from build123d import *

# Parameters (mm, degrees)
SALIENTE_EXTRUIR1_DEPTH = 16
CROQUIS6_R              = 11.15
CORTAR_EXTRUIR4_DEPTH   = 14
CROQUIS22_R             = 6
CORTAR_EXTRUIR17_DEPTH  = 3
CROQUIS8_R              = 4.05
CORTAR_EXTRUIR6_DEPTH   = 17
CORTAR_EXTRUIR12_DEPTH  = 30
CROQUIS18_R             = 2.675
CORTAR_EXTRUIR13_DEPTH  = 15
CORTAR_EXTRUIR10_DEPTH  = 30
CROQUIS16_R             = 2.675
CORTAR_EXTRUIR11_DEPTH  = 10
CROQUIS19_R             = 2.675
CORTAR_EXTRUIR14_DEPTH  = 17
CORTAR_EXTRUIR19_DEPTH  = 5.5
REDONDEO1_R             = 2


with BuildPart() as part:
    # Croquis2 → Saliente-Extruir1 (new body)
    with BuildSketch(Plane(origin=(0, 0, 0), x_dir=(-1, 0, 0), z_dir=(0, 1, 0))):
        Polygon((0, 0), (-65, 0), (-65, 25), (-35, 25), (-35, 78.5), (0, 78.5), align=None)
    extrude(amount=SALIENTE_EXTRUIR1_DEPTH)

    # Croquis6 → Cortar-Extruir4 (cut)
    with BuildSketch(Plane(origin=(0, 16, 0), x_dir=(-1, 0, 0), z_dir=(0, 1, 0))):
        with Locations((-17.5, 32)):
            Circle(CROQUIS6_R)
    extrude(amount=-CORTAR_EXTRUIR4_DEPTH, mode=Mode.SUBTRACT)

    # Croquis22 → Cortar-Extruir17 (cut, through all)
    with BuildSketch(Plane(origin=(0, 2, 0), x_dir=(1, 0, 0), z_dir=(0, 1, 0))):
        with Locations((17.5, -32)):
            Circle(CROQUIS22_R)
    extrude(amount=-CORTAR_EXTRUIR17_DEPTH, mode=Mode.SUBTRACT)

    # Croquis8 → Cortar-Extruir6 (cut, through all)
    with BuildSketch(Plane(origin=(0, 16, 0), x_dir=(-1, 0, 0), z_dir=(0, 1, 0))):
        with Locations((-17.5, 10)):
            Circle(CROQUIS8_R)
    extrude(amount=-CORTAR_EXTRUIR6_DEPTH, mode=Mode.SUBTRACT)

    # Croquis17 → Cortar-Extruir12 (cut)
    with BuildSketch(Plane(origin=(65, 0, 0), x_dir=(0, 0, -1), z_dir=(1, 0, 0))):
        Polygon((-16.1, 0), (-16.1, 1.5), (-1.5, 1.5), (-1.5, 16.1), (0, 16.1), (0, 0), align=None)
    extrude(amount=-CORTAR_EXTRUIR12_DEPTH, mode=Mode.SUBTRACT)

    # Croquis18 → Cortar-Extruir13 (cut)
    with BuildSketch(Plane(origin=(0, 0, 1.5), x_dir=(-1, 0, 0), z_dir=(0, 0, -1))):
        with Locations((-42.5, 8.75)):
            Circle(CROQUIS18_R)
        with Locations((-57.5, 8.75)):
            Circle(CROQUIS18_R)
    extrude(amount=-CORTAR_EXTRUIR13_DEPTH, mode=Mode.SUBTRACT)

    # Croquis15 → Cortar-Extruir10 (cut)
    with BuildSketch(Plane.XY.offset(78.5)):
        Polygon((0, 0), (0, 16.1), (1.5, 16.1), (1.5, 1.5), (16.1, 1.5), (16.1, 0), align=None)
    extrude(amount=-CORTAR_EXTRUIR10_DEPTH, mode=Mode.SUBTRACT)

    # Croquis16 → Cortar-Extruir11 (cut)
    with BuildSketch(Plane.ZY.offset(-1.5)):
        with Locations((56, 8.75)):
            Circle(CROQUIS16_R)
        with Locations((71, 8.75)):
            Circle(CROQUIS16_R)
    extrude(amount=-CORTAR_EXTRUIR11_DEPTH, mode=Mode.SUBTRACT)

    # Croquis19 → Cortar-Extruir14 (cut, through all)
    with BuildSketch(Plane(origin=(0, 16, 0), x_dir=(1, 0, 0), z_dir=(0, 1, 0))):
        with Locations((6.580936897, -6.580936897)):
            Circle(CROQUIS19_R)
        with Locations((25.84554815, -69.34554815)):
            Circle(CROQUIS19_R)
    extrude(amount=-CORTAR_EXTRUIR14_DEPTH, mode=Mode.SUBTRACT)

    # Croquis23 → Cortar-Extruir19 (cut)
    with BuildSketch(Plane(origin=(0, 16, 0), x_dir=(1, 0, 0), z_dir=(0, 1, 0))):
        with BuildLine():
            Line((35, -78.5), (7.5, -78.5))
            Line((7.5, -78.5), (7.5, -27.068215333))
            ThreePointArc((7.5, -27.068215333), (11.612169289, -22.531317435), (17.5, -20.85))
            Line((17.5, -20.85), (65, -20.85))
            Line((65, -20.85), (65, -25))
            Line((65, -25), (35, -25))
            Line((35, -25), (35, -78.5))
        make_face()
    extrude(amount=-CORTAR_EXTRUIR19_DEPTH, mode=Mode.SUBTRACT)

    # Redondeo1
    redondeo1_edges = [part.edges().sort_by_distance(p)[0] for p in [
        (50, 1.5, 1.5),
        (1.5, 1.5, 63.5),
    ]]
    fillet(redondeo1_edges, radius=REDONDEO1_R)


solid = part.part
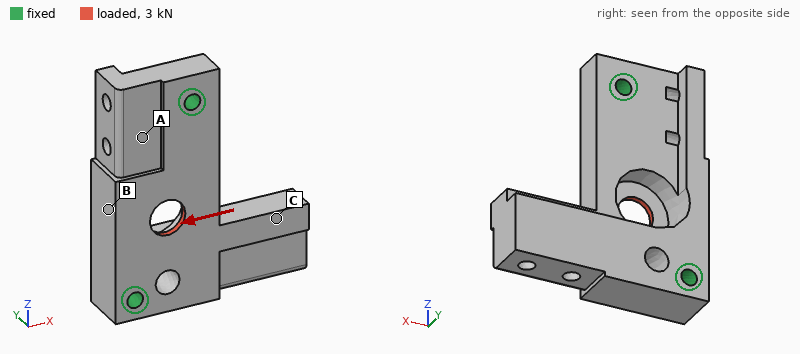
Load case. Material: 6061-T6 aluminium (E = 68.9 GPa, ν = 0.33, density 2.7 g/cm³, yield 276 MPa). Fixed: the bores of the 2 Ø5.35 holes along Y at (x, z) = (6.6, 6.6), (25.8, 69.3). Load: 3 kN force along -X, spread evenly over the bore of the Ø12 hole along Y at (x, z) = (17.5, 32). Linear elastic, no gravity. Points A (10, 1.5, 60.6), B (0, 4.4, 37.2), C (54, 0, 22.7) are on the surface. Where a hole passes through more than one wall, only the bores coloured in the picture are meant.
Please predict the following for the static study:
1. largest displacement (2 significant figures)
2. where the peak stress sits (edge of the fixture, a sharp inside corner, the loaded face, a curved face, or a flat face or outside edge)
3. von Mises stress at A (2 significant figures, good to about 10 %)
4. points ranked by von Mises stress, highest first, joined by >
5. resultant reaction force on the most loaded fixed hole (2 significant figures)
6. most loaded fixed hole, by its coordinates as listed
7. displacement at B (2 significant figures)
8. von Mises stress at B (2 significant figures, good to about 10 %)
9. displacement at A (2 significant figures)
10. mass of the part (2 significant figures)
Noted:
32 µm
the loaded face
10 MPa
B > A > C
1.7 kN
(6.6, 6.6)
13 µm
20 MPa
7.2 µm
100 g
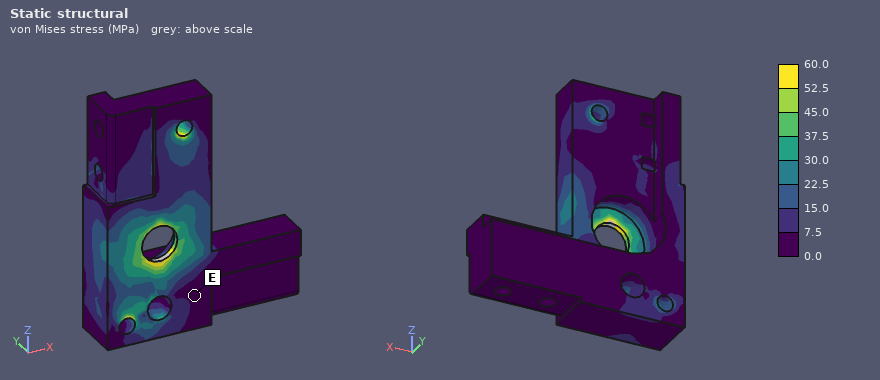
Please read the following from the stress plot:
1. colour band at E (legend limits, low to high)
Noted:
0.0 to 7.5 MPa
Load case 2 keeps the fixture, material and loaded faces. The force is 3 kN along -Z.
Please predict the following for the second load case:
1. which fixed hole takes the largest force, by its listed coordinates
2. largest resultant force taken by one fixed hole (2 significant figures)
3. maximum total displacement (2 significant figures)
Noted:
(6.6, 6.6)
1.6 kN
12 µm
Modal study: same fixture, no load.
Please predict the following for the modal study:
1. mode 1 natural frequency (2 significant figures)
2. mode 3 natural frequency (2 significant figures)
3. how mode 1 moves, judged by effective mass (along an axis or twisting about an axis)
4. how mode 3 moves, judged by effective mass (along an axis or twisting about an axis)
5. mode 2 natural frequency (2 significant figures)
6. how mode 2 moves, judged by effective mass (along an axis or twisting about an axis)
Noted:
3300 Hz
9900 Hz
along Y
along Y
6700 Hz
along Z
